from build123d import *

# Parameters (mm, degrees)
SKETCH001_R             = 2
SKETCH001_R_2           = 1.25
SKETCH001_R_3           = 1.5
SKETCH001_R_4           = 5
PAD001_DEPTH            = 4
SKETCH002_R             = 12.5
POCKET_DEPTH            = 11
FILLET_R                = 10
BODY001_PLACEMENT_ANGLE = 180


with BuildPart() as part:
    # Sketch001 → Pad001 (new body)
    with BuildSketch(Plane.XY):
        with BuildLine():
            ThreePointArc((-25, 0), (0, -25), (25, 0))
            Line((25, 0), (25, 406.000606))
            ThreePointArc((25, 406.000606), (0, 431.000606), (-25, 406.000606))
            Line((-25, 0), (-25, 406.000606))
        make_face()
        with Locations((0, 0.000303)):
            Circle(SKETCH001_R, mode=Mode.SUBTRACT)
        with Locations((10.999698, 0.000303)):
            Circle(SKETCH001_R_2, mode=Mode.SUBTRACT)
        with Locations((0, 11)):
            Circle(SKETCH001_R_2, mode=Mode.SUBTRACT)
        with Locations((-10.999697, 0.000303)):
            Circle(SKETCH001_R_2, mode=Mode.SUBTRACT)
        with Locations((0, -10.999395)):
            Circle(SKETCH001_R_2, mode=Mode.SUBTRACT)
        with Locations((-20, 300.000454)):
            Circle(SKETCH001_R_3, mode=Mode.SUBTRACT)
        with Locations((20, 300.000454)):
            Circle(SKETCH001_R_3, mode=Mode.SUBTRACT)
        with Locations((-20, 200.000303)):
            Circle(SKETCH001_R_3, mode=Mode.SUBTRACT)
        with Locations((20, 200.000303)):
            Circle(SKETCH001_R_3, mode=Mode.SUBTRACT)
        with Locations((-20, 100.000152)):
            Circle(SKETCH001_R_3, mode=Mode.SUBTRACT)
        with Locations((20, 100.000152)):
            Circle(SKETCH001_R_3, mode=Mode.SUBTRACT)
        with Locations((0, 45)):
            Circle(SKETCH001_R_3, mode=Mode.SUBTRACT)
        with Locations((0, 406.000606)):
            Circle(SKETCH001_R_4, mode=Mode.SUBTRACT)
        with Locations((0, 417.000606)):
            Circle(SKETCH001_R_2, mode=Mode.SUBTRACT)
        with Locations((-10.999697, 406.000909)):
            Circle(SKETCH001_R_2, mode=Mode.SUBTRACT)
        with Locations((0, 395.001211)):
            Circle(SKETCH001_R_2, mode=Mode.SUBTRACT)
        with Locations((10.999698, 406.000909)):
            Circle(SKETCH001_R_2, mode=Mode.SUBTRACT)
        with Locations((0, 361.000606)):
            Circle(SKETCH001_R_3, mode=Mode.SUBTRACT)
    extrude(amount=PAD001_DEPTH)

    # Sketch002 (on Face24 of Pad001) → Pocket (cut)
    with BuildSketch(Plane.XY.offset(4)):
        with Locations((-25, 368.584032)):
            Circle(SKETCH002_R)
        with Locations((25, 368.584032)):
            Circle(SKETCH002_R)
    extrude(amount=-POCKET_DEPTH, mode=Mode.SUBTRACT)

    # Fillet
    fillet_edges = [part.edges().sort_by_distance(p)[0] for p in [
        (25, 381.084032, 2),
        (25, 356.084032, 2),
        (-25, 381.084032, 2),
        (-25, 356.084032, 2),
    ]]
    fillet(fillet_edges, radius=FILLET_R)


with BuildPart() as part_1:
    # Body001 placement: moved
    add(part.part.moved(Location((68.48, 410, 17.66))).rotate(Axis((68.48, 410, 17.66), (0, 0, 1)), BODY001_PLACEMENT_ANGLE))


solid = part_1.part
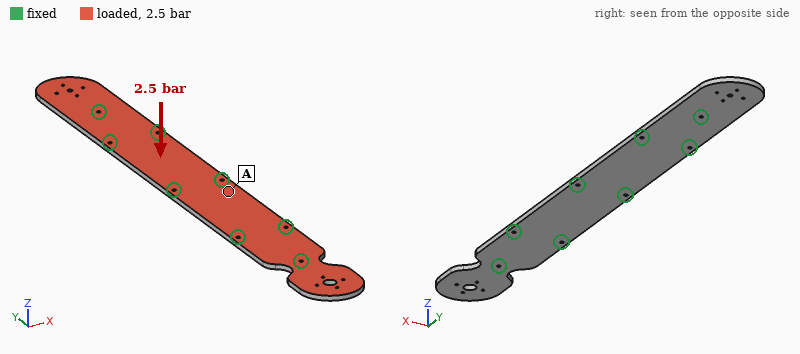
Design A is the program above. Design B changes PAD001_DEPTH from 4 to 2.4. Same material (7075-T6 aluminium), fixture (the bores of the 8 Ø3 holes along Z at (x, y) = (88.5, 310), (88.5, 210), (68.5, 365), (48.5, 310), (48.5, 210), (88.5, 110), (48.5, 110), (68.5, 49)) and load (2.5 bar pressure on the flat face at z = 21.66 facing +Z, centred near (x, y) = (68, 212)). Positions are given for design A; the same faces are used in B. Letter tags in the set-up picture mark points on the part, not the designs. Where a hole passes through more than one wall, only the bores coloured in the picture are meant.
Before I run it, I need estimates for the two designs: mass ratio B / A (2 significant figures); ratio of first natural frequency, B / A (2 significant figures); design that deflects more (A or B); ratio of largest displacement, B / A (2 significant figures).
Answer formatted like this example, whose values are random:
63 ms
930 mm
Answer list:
0.60
0.61
B
4.4
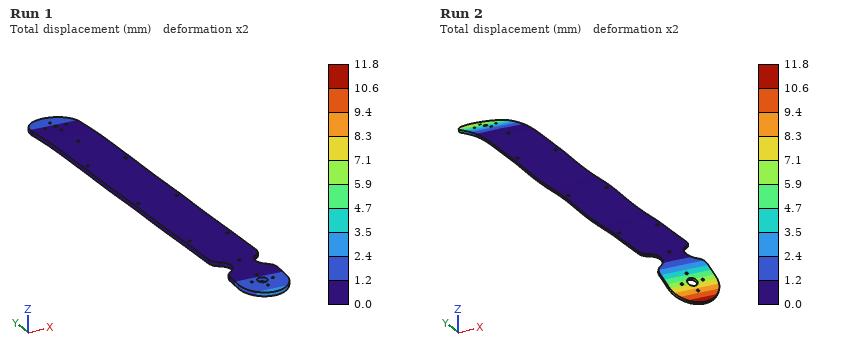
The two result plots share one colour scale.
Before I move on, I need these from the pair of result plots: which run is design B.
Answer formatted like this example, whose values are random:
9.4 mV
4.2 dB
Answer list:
Run 2
